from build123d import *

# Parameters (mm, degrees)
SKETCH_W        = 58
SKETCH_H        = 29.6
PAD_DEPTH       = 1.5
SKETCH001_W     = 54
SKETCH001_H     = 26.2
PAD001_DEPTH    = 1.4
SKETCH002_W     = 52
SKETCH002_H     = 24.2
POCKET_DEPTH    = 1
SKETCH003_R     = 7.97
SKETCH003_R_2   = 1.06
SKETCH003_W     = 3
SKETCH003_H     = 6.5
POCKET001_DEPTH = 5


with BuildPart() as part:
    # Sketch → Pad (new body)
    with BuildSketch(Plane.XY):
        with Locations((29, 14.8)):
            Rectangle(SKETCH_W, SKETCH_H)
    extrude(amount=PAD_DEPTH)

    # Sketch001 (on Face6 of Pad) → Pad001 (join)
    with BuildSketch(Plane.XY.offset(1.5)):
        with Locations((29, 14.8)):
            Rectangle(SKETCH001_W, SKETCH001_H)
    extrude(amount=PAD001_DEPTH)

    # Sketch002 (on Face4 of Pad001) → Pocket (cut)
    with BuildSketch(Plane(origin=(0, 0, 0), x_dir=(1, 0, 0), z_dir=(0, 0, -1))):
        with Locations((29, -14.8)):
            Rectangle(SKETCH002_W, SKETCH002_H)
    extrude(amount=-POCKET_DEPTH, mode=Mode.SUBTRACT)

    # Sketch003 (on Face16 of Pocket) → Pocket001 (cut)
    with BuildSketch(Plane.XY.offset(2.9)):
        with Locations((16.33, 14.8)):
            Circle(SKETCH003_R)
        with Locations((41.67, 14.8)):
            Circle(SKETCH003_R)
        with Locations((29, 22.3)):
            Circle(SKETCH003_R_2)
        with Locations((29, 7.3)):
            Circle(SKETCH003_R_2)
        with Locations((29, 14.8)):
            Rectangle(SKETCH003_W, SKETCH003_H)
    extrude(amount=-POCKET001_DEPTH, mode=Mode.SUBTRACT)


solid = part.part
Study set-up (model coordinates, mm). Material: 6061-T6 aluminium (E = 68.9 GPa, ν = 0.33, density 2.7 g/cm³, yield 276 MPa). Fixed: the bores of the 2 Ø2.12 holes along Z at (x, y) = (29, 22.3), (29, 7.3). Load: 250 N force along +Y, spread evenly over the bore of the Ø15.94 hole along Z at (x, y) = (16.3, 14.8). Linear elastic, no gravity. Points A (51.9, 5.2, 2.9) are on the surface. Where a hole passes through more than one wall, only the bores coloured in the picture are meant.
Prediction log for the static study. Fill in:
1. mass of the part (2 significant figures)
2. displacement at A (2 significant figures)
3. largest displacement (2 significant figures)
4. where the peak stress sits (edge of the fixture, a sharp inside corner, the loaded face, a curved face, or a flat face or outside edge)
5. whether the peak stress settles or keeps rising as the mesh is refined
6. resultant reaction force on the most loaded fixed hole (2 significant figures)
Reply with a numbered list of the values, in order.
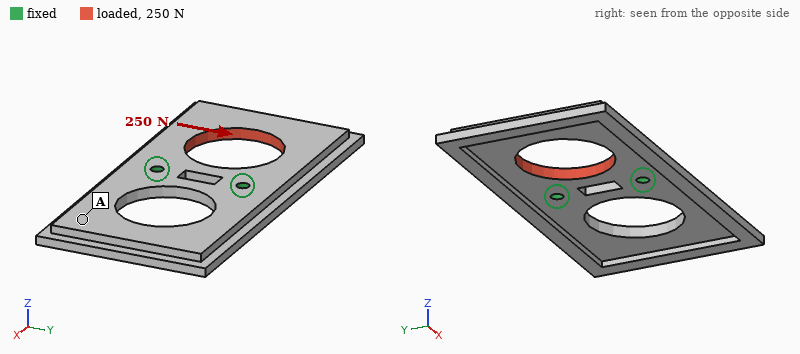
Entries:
1. 6.7 g
2. 9.8 µm
3. 28 µm
4. edge of the fixture
5. keeps rising
6. 200 N
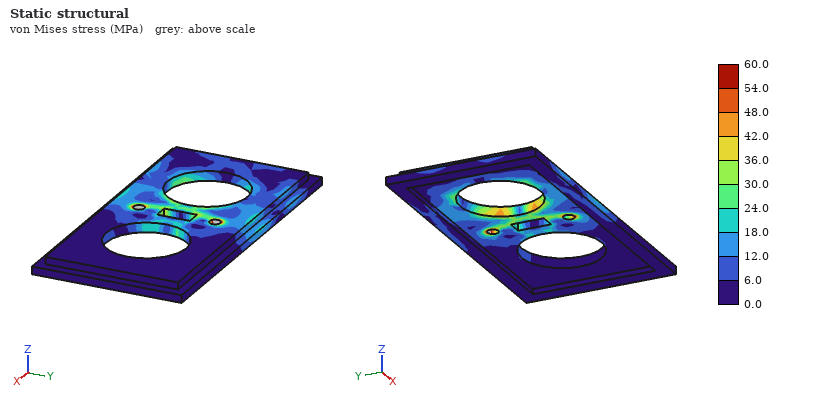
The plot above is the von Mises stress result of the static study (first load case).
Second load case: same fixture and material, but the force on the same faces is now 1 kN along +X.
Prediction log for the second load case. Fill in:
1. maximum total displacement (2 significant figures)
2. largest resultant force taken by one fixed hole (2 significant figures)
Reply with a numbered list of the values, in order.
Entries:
1. 30 µm
2. 500 N
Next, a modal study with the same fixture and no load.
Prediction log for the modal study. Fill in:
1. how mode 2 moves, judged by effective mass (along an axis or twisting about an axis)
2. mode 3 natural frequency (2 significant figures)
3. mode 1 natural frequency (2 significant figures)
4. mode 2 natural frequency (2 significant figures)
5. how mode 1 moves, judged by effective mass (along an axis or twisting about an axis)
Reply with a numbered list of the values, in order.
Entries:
1. along Z
2. 3500 Hz
3. 1700 Hz
4. 2000 Hz
5. twisting about Y
